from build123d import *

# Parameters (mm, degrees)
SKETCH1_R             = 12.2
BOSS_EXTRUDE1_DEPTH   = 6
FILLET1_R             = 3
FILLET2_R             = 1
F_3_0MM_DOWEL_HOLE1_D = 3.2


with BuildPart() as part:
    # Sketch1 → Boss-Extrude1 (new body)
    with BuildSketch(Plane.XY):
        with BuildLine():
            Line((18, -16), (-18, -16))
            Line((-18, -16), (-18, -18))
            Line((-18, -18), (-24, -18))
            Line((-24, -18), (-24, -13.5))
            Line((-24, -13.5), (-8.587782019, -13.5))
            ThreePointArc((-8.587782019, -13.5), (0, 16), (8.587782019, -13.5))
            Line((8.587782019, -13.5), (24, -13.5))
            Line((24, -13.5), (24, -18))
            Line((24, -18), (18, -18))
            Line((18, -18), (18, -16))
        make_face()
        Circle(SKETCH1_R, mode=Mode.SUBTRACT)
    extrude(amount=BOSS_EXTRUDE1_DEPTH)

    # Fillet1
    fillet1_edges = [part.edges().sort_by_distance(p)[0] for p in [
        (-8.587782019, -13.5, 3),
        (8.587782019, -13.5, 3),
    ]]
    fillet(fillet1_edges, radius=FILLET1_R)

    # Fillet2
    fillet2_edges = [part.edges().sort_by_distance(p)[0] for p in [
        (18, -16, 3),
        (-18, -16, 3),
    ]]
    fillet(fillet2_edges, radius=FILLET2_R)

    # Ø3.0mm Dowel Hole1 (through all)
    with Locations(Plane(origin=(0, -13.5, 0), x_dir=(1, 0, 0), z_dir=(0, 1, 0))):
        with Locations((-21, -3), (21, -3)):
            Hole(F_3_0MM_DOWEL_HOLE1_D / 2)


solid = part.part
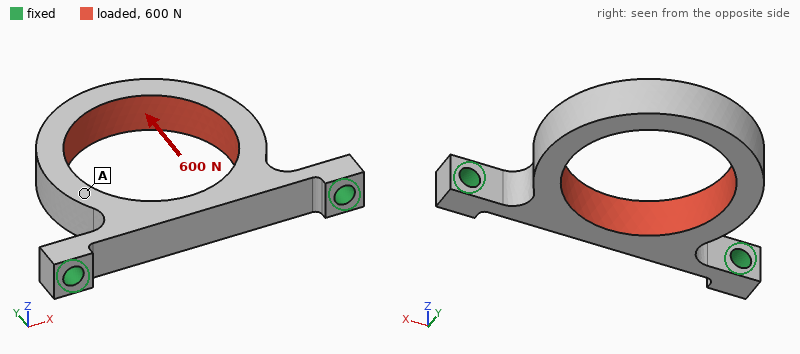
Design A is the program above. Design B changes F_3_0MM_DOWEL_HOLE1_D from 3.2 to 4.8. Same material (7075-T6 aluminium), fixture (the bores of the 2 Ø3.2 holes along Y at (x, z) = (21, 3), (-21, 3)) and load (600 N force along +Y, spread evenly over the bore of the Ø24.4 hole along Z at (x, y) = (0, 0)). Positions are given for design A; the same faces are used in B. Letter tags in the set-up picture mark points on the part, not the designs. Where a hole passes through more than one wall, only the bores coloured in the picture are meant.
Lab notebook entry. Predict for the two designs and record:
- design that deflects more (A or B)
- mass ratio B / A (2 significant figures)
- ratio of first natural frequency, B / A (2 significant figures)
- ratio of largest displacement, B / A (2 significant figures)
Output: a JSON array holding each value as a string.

["A", "0.97", "1.0", "0.92"]
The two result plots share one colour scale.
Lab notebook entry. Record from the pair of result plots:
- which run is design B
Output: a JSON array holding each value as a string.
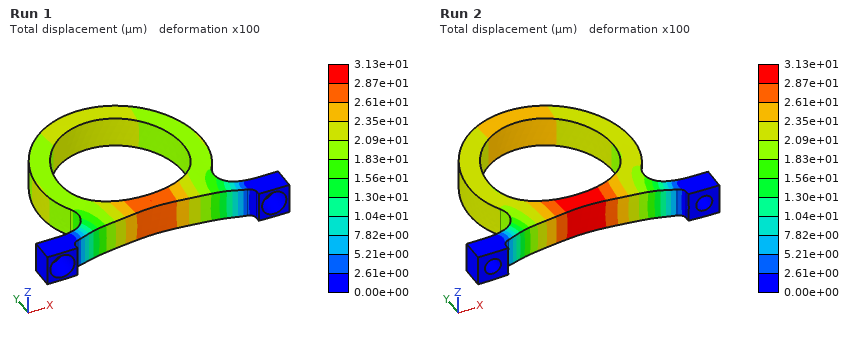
["Run 1"]
